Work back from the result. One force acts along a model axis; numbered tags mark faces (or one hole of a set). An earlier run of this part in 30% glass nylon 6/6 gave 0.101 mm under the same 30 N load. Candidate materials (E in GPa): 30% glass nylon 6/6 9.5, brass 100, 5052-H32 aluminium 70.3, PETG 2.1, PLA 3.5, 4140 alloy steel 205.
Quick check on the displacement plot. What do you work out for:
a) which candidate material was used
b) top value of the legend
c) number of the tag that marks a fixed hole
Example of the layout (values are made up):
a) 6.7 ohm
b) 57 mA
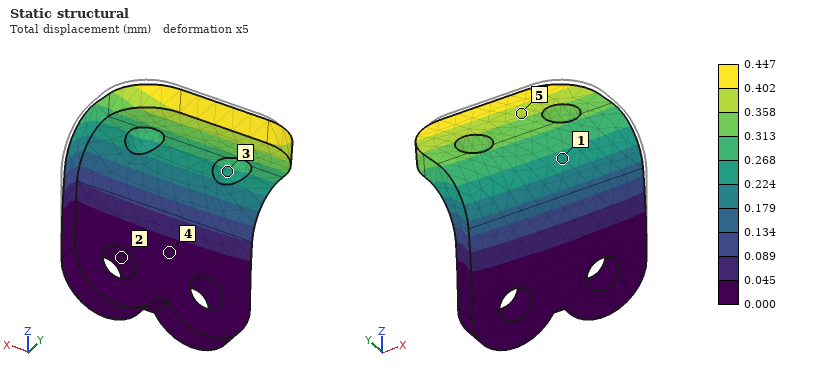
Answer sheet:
a) PETG
b) 0.447 mm
c) 2
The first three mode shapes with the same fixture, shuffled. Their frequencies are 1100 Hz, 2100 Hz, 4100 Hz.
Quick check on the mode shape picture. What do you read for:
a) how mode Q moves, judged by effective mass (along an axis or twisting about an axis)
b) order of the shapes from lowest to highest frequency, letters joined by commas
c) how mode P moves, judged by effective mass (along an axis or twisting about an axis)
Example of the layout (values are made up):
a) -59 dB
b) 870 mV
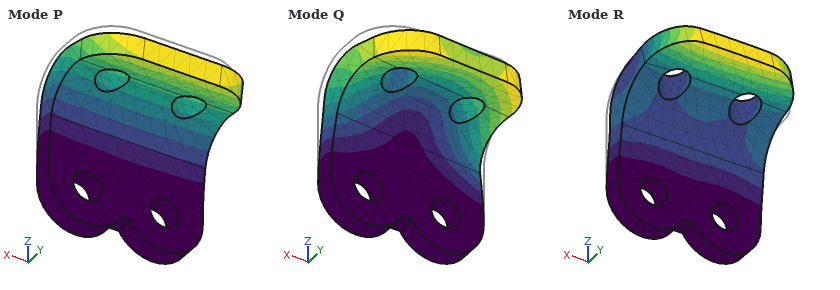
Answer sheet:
a) along X
b) P, Q, R
c) along Y
